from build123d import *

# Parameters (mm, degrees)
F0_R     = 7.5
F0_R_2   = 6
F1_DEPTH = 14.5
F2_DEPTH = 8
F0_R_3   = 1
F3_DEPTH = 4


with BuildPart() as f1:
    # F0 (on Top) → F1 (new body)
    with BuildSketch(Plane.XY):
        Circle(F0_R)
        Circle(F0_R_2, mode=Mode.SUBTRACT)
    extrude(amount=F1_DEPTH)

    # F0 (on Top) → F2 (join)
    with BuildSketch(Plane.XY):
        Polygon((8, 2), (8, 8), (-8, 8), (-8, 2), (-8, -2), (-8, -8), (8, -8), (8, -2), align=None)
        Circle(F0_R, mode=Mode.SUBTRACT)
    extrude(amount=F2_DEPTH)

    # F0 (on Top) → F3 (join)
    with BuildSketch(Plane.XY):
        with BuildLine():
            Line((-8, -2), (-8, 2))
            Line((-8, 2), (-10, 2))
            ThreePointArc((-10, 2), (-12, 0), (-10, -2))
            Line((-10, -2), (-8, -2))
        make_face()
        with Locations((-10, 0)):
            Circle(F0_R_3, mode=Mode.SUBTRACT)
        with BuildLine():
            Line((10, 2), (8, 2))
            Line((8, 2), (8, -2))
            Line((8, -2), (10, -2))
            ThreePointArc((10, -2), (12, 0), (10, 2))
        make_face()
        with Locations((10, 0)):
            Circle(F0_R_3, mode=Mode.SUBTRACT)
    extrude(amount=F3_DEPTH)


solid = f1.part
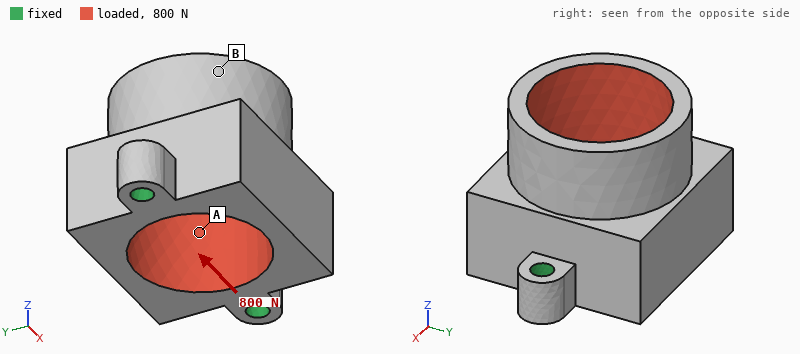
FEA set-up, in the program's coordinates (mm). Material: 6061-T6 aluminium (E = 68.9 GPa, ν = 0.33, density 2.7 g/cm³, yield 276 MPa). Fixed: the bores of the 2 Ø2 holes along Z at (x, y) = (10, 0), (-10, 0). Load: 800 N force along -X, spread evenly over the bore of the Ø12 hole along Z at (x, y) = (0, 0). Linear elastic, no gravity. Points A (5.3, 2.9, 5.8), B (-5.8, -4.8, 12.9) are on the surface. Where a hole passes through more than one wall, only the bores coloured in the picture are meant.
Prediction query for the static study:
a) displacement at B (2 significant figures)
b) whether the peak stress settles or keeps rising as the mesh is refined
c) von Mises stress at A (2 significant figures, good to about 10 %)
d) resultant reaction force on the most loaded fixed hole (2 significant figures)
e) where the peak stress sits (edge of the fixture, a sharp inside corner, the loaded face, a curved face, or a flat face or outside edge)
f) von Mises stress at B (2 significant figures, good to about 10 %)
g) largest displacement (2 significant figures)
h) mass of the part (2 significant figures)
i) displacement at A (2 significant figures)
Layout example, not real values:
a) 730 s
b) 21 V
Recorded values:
a) 8.4 µm
b) keeps rising
c) 23 MPa
d) 460 N
e) a sharp inside corner
f) 6.6 MPa
g) 9.1 µm
h) 4.4 g
i) 4.1 µm
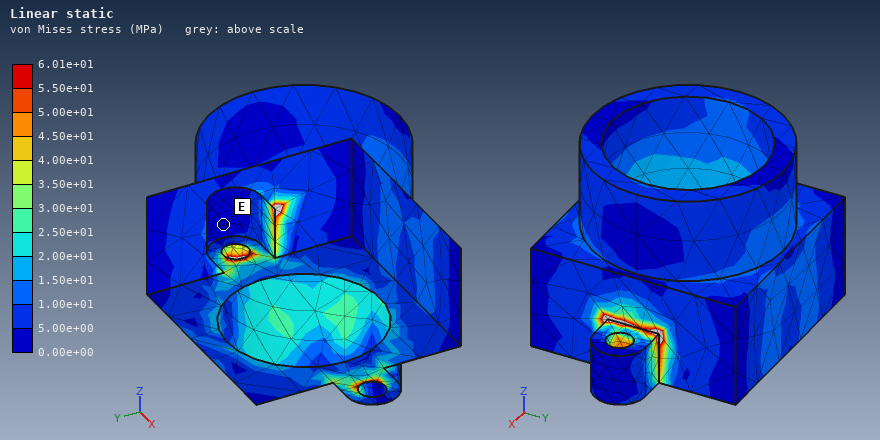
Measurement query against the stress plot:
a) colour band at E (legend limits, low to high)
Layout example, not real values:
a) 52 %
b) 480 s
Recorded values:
a) 0.00e+00 to 5.00e+00 MPa
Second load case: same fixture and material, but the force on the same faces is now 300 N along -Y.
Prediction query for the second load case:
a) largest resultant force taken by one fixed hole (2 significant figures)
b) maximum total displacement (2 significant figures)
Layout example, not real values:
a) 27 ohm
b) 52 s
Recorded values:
a) 150 N
b) 29 µm
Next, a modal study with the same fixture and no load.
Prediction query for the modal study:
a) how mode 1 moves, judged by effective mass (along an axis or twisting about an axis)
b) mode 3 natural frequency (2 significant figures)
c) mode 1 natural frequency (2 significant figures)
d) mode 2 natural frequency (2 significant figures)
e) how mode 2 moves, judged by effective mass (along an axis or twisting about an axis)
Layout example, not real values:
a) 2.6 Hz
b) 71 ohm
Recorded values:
a) along Y
b) 27 kHz
c) 9300 Hz
d) 26 kHz
e) along Z
